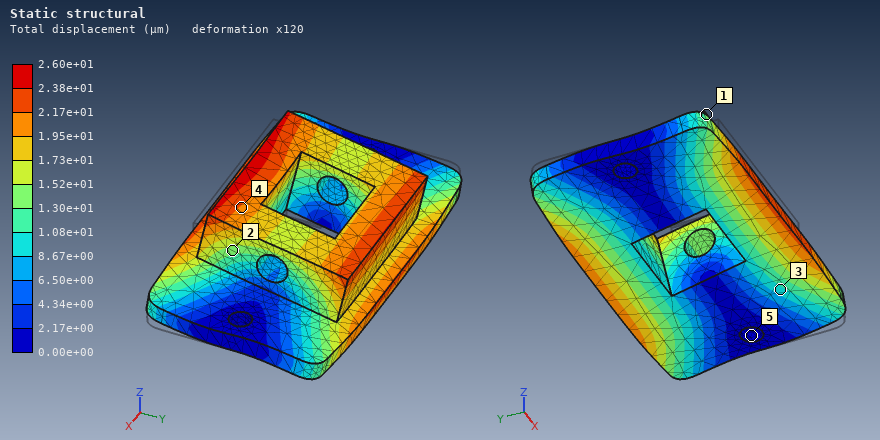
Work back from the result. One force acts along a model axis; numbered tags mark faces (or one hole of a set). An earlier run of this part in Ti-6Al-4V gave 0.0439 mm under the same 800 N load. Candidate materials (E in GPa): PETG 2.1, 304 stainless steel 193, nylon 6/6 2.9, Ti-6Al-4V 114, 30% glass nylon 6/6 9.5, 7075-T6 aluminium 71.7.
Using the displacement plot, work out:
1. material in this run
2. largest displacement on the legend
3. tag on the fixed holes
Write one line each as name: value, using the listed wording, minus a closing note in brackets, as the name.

material in this run: 304 stainless steel
largest displacement on the legend: 2.60e+01 µm
tag on the fixed holes: 5
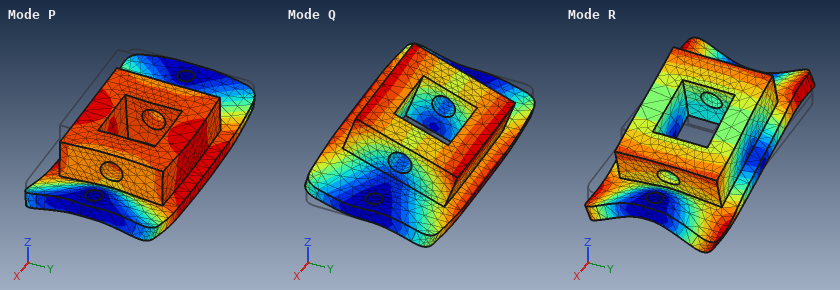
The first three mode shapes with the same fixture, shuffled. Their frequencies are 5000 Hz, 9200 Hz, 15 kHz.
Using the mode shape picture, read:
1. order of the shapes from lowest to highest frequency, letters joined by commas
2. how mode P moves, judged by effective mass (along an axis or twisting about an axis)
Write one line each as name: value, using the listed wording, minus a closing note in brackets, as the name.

order of the shapes from lowest to highest frequency, letters joined by commas: Q, P, R
how mode P moves, judged by effective mass: along Z
